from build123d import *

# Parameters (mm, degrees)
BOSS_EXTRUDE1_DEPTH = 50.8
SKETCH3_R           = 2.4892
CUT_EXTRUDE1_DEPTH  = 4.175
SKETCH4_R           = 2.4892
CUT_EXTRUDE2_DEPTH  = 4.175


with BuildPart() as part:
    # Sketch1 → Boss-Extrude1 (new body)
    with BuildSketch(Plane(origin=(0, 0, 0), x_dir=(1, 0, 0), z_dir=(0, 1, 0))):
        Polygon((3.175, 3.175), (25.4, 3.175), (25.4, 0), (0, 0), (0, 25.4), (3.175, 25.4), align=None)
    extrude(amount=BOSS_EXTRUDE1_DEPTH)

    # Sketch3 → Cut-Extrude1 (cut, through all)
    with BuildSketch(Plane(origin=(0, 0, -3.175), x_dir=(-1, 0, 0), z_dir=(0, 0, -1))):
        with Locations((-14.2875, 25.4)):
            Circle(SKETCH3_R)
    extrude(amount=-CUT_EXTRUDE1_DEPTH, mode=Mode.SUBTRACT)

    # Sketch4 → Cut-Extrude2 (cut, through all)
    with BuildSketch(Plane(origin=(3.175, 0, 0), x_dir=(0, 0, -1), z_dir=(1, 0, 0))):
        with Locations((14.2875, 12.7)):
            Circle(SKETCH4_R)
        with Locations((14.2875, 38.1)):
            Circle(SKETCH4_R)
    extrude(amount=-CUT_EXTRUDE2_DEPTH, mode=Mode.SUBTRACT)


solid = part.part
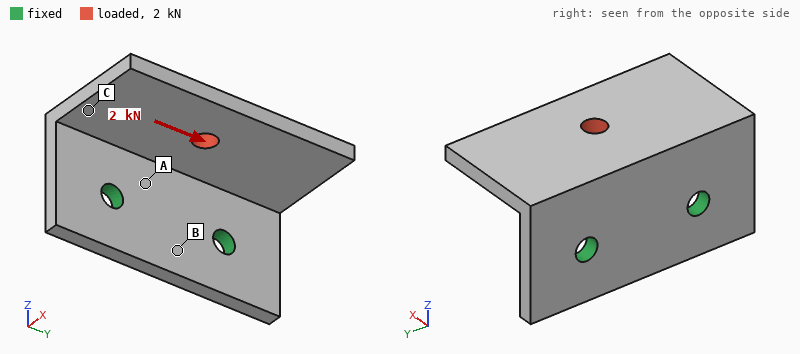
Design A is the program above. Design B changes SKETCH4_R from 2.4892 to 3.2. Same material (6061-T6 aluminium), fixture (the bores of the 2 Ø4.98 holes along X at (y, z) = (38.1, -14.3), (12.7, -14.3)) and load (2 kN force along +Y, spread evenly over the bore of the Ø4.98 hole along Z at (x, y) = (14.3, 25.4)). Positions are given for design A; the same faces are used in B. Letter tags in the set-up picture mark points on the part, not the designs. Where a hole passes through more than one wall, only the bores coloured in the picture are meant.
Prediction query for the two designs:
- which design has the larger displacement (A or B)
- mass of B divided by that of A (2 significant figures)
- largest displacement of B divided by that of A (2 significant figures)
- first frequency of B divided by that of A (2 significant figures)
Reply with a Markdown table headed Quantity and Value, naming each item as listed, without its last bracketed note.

| Quantity | Value |
|---|---|
| which design has the larger displacement | A |
| mass of B divided by that of A | 0.99 |
| largest displacement of B divided by that of A | 0.87 |
| first frequency of B divided by that of A | 1.0 |
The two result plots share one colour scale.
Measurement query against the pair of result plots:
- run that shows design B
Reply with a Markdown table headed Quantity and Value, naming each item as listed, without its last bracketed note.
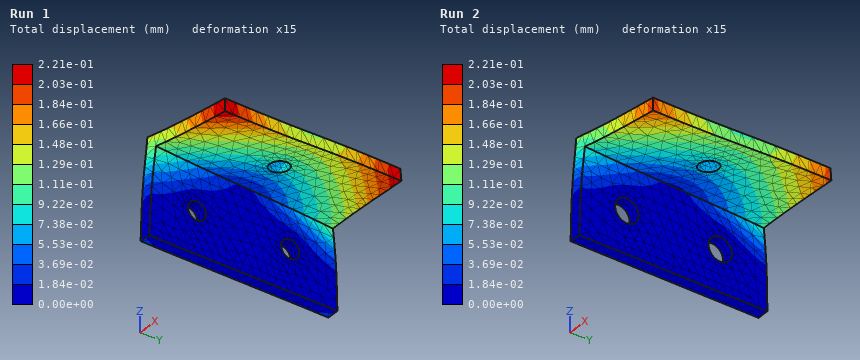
| Quantity | Value |
|---|---|
| run that shows design B | Run 2 |
